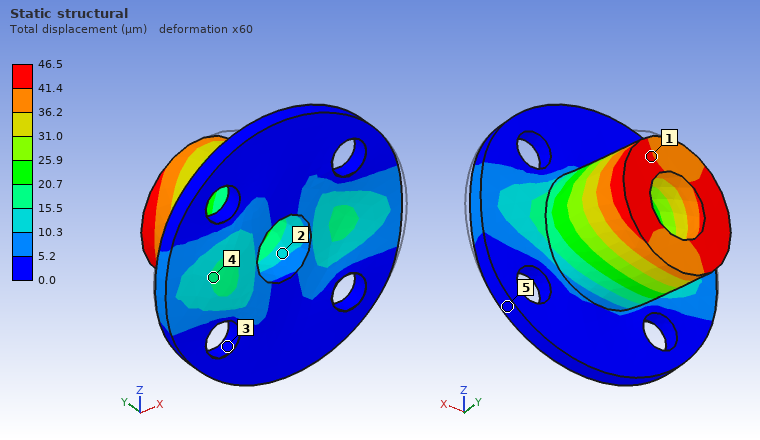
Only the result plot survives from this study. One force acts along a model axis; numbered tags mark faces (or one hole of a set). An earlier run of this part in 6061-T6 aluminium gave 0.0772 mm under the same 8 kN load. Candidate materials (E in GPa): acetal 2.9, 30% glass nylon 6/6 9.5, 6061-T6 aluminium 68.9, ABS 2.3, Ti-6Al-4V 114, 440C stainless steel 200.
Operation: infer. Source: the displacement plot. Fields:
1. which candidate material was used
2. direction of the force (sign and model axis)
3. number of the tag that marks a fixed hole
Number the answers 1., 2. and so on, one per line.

1. Ti-6Al-4V
2. -X
3. 3
